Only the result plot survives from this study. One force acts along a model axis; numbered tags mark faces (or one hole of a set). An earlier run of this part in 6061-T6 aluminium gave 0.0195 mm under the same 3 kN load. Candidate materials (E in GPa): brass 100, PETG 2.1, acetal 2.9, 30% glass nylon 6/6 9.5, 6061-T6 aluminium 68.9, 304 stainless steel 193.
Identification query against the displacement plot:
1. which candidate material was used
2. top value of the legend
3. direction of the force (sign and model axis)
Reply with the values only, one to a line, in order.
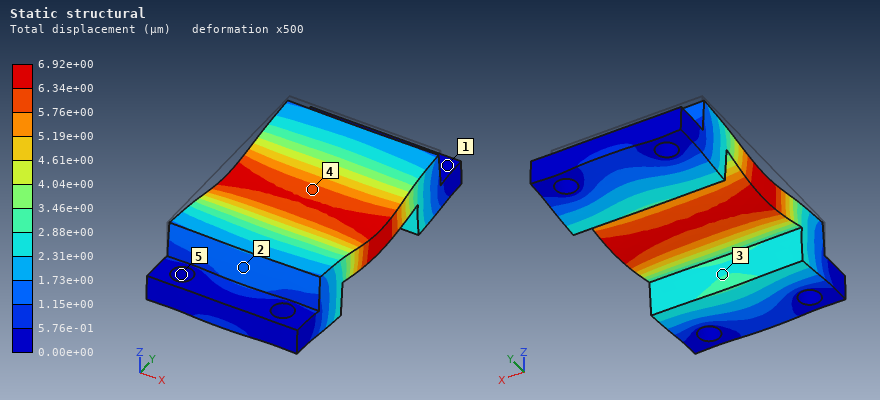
304 stainless steel
6.92e+00 µm
-Z
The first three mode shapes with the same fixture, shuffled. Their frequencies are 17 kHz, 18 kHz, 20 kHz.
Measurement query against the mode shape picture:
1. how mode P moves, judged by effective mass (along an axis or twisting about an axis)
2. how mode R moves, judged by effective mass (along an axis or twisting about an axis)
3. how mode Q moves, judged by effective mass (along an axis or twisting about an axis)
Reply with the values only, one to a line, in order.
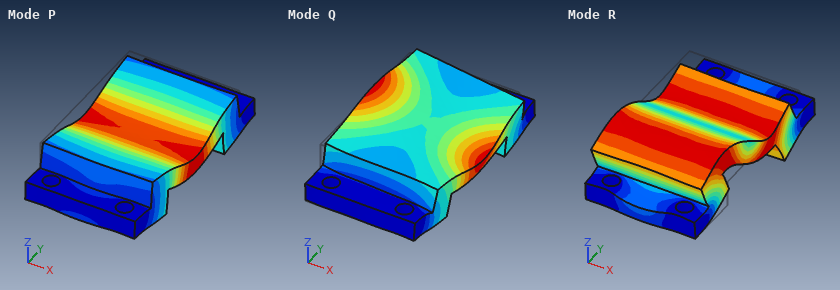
along Z
along Y
along X
